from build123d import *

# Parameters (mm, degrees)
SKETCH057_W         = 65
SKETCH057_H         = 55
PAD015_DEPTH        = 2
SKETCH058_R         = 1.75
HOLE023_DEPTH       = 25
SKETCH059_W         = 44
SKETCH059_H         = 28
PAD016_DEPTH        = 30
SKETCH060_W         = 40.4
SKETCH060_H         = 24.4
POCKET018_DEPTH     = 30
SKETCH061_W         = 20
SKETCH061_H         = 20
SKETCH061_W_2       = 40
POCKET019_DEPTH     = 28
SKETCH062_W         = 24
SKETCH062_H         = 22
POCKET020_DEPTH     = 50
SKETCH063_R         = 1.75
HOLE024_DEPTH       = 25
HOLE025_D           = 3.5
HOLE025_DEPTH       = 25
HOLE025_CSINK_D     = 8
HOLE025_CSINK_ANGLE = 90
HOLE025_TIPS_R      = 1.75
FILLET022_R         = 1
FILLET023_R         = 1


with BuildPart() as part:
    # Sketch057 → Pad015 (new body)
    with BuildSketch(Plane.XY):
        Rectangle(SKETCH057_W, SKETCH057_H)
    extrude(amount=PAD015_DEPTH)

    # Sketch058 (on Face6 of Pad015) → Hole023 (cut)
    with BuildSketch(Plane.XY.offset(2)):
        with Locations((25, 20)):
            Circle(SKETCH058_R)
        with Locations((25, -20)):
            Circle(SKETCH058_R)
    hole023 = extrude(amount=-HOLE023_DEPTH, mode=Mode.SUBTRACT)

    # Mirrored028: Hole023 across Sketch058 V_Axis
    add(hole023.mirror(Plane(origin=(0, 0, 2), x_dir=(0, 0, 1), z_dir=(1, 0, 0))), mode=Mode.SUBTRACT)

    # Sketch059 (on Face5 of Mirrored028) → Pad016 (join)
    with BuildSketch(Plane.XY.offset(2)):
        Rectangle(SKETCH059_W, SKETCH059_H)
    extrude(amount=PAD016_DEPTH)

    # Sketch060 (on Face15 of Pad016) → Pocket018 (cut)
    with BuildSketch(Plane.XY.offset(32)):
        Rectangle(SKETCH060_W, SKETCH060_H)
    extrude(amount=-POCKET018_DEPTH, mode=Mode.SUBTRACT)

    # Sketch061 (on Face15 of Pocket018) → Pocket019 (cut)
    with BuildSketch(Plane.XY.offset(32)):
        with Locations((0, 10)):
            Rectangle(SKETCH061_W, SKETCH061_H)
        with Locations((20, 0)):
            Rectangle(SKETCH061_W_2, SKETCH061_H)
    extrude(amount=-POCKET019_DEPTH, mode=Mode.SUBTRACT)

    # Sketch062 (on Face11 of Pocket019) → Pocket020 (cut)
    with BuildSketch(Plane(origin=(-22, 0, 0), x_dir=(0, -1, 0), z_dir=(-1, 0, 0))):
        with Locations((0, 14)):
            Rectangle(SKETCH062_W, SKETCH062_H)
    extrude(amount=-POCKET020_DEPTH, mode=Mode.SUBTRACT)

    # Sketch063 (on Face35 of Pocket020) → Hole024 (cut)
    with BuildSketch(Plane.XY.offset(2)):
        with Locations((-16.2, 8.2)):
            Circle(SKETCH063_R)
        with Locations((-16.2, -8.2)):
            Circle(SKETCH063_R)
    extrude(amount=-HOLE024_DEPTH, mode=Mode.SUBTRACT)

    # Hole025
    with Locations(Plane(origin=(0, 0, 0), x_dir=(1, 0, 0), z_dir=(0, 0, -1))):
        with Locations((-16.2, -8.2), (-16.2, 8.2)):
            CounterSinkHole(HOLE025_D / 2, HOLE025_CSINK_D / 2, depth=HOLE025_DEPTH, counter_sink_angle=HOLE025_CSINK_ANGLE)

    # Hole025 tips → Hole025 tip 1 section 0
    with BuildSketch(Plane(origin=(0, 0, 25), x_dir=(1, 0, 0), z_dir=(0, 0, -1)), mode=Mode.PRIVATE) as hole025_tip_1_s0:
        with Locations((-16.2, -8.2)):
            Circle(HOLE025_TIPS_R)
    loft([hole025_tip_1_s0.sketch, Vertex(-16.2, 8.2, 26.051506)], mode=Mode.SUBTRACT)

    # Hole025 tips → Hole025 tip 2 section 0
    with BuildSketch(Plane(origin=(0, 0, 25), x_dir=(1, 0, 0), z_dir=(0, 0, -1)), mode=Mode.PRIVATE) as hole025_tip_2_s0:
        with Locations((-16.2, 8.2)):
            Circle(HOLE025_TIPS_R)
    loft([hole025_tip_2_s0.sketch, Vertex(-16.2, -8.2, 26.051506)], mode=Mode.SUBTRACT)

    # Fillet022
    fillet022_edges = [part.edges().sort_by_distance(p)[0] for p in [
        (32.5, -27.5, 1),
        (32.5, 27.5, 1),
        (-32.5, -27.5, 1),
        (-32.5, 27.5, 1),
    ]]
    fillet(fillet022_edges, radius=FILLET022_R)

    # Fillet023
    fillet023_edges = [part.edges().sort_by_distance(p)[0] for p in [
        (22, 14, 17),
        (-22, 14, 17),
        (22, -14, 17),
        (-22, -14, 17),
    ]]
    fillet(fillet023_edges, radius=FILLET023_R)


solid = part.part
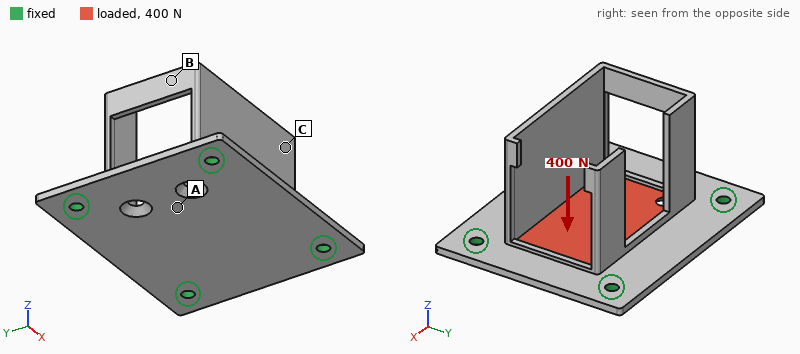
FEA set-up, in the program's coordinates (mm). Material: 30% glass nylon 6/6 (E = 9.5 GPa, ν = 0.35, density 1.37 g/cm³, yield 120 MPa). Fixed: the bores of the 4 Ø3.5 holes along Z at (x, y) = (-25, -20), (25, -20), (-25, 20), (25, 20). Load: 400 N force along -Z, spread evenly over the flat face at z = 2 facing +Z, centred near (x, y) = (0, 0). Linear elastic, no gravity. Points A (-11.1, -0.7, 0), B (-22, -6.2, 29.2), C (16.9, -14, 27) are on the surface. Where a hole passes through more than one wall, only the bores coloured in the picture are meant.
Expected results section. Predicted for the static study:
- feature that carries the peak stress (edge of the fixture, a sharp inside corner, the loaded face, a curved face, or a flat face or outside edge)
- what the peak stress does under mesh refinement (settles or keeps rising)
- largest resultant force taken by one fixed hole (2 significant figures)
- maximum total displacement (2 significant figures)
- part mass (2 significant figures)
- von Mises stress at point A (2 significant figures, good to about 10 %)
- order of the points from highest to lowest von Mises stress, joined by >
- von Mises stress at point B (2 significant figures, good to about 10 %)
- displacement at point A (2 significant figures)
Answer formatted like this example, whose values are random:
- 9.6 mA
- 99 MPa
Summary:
- edge of the fixture
- keeps rising
- 120 N
- 0.89 mm
- 15 g
- 29 MPa
- A > B > C
- 16 MPa
- 0.41 mm
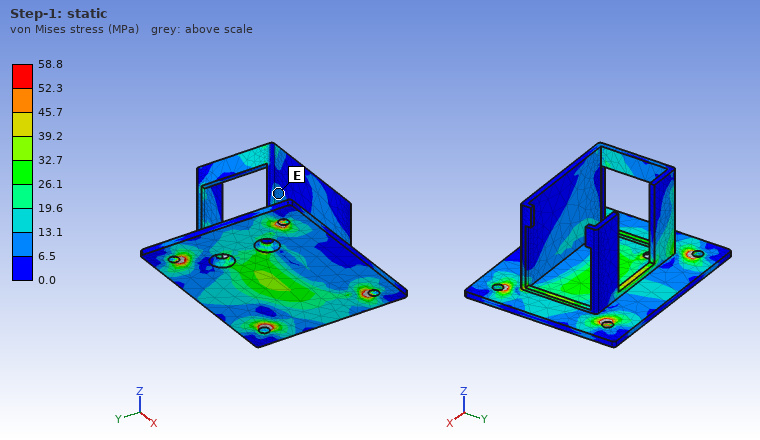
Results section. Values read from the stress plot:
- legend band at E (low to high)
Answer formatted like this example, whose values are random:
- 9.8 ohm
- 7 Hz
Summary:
- 6.5 to 13.1 MPa
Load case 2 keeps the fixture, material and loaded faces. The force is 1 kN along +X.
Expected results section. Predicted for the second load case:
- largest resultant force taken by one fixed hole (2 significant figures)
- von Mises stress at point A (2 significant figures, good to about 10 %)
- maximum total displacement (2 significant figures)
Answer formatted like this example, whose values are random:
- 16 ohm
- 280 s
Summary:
- 270 N
- 3.0 MPa
- 59 µm
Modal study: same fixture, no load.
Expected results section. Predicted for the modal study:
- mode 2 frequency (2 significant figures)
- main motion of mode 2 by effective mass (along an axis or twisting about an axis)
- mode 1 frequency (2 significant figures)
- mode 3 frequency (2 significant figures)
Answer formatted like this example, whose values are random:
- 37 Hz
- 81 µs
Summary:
- 920 Hz
- along Y
- 770 Hz
- 1300 Hz
